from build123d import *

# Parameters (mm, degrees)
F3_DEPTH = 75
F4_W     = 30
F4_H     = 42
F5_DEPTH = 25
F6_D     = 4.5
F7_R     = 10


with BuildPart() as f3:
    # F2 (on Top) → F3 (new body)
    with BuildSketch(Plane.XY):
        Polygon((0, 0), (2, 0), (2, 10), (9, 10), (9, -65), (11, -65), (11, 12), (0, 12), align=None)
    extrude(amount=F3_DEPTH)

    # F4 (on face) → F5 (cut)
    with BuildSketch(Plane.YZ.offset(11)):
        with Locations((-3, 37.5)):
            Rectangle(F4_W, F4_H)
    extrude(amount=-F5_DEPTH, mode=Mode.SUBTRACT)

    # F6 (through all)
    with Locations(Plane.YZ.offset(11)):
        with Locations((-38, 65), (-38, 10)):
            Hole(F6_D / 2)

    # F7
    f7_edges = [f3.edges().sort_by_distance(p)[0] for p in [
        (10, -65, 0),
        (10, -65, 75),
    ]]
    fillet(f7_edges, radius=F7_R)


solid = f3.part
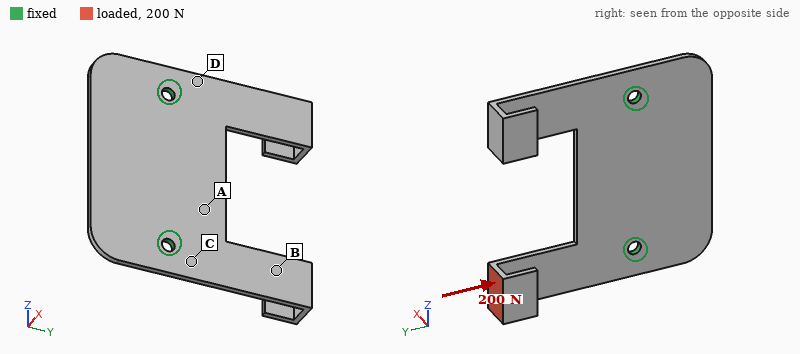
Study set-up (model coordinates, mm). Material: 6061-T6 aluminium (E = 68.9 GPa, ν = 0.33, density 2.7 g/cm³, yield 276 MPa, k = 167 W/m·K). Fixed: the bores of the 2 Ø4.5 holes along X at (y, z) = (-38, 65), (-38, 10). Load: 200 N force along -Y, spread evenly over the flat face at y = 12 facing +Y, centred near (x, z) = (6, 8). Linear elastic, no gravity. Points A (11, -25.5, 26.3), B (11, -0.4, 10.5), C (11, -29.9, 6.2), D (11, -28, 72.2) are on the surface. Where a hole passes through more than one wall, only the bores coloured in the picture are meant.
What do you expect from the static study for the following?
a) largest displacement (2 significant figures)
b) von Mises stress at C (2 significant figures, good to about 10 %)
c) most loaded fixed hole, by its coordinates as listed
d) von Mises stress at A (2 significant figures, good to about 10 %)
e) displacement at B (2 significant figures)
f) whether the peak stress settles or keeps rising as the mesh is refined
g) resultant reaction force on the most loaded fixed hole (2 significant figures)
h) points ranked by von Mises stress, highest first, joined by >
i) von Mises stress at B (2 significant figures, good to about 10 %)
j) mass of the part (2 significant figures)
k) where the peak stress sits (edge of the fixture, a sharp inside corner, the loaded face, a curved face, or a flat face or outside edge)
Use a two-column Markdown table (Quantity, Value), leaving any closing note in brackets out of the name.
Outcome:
| Quantity | Value |
|---|---|
| largest displacement | 1.2 mm |
| von Mises stress at C | 43 MPa |
| most loaded fixed hole, by its coordinates as listed | (-38, 10) |
| von Mises stress at A | 24 MPa |
| displacement at B | 0.58 mm |
| whether the peak stress settles or keeps rising as the mesh is refined | keeps rising |
| resultant reaction force on the most loaded fixed hole | 200 N |
| points ranked by von Mises stress, highest first, joined by > | B > C > A > D |
| von Mises stress at B | 72 MPa |
| mass of the part | 27 g |
| where the peak stress sits | a sharp inside corner |
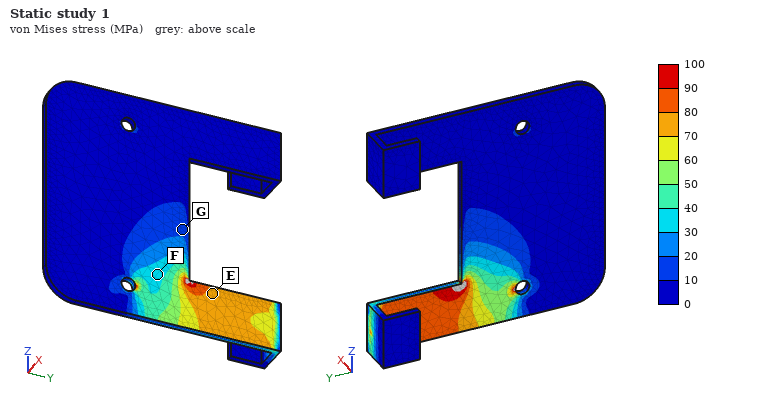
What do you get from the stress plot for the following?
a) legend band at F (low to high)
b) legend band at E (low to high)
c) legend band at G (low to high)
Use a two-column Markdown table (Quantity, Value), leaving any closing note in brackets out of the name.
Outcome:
| Quantity | Value |
|---|---|
| legend band at F | 30 to 40 MPa |
| legend band at E | 70 to 80 MPa |
| legend band at G | 10 to 20 MPa |
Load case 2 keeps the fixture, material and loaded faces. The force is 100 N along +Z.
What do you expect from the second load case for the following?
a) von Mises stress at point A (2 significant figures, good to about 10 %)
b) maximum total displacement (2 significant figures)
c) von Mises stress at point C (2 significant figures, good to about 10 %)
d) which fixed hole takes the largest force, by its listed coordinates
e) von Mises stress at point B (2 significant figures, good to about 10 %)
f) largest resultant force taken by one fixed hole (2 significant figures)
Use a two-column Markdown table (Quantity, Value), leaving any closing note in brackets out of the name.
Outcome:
| Quantity | Value |
|---|---|
| von Mises stress at point A | 7.6 MPa |
| maximum total displacement | 0.27 mm |
| von Mises stress at point C | 30 MPa |
| which fixed hole takes the largest force, by its listed coordinates | (-38, 65) |
| von Mises stress at point B | 30 MPa |
| largest resultant force taken by one fixed hole | 110 N |
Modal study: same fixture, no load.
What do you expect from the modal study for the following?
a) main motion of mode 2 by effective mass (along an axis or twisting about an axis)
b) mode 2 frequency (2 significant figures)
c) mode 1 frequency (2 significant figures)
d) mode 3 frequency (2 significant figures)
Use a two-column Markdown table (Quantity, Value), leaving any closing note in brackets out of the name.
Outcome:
| Quantity | Value |
|---|---|
| main motion of mode 2 by effective mass | twisting about Y |
| mode 2 frequency | 540 Hz |
| mode 1 frequency | 520 Hz |
| mode 3 frequency | 1800 Hz |
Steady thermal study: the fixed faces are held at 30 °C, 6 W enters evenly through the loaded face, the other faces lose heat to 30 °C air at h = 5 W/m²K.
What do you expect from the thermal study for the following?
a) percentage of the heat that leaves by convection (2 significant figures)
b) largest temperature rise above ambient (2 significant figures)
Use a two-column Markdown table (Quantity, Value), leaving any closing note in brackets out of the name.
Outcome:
| Quantity | Value |
|---|---|
| percentage of the heat that leaves by convection | 6.6 % |
| largest temperature rise above ambient | 49 K |
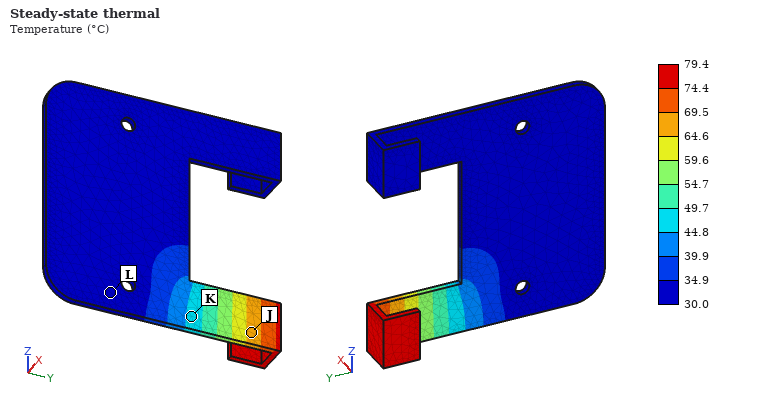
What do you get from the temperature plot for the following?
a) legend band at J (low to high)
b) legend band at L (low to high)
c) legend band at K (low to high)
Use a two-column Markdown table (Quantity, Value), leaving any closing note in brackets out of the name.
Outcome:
| Quantity | Value |
|---|---|
| legend band at J | 64.6 to 69.5 °C |
| legend band at L | 30.0 to 34.9 °C |
| legend band at K | 44.8 to 49.7 °C |
